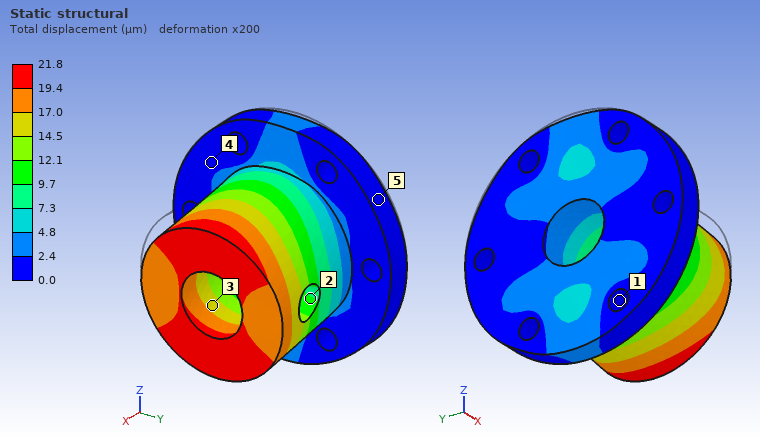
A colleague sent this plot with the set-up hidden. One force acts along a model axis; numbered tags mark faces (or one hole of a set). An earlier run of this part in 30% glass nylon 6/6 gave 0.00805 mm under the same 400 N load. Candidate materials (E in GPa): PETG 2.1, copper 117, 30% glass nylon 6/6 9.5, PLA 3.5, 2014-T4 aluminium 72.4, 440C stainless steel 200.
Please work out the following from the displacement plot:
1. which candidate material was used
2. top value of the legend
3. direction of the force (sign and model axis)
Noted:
PLA
21.8 µm
-Z
